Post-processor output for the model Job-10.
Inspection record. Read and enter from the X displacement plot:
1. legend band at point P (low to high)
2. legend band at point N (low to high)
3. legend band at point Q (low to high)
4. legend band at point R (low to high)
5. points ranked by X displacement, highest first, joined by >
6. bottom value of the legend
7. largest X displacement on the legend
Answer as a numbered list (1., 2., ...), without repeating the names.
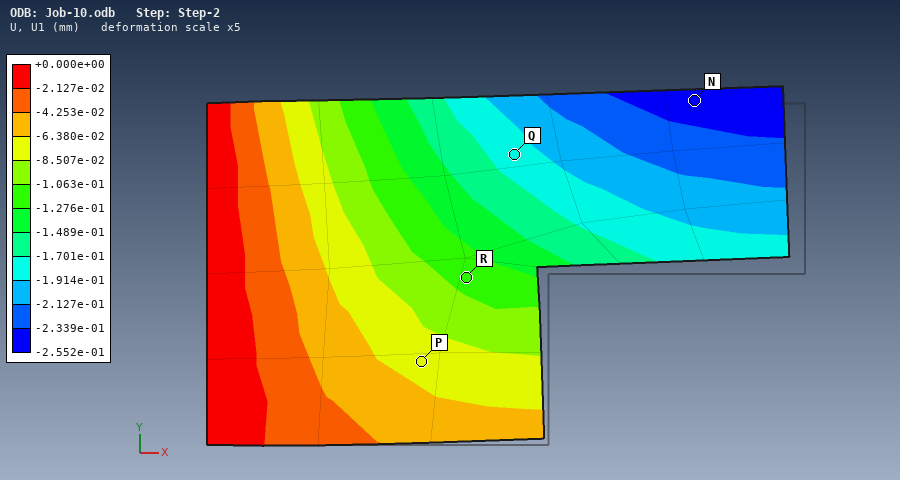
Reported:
1. -8.507e-02 to -6.380e-02 mm
2. -2.552e-01 to -2.339e-01 mm
3. -1.914e-01 to -1.701e-01 mm
4. -1.276e-01 to -1.063e-01 mm
5. P > R > Q > N
6. -2.552e-01 mm
7. +0.000e+00 mm
